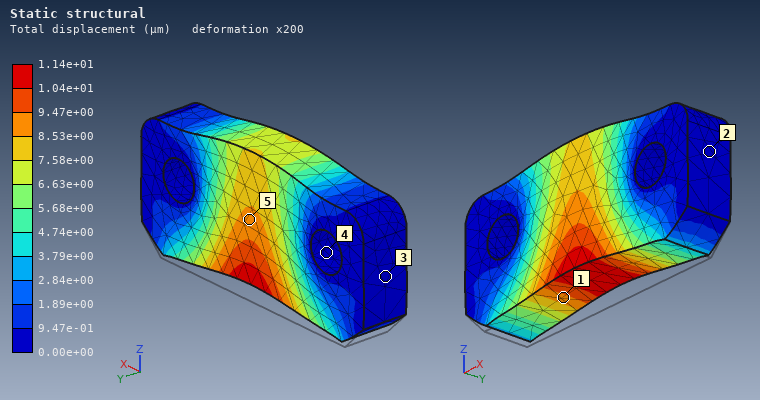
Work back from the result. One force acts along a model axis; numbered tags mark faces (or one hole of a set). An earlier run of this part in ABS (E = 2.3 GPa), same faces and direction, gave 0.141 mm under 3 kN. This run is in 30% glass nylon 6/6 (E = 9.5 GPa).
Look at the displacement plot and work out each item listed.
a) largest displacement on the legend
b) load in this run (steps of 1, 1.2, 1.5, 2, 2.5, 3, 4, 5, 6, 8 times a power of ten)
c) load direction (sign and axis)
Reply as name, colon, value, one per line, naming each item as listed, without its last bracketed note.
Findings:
largest displacement on the legend: 1.14e+01 µm
load in this run: 1 kN
load direction: +Z
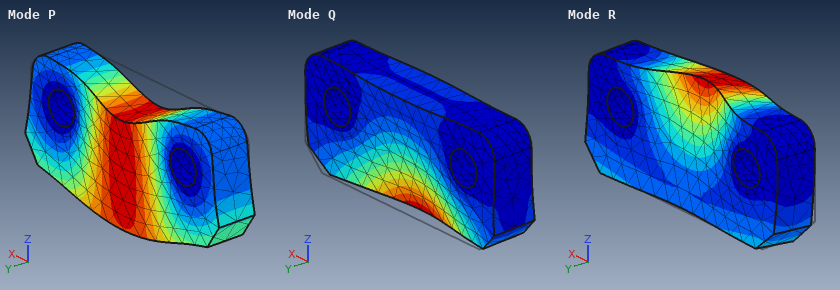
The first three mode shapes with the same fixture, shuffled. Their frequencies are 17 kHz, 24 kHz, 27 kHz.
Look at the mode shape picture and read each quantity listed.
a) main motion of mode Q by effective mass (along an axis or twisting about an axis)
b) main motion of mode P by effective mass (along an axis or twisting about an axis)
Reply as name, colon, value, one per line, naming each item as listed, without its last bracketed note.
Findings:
main motion of mode Q by effective mass: along Y
main motion of mode P by effective mass: along Z
